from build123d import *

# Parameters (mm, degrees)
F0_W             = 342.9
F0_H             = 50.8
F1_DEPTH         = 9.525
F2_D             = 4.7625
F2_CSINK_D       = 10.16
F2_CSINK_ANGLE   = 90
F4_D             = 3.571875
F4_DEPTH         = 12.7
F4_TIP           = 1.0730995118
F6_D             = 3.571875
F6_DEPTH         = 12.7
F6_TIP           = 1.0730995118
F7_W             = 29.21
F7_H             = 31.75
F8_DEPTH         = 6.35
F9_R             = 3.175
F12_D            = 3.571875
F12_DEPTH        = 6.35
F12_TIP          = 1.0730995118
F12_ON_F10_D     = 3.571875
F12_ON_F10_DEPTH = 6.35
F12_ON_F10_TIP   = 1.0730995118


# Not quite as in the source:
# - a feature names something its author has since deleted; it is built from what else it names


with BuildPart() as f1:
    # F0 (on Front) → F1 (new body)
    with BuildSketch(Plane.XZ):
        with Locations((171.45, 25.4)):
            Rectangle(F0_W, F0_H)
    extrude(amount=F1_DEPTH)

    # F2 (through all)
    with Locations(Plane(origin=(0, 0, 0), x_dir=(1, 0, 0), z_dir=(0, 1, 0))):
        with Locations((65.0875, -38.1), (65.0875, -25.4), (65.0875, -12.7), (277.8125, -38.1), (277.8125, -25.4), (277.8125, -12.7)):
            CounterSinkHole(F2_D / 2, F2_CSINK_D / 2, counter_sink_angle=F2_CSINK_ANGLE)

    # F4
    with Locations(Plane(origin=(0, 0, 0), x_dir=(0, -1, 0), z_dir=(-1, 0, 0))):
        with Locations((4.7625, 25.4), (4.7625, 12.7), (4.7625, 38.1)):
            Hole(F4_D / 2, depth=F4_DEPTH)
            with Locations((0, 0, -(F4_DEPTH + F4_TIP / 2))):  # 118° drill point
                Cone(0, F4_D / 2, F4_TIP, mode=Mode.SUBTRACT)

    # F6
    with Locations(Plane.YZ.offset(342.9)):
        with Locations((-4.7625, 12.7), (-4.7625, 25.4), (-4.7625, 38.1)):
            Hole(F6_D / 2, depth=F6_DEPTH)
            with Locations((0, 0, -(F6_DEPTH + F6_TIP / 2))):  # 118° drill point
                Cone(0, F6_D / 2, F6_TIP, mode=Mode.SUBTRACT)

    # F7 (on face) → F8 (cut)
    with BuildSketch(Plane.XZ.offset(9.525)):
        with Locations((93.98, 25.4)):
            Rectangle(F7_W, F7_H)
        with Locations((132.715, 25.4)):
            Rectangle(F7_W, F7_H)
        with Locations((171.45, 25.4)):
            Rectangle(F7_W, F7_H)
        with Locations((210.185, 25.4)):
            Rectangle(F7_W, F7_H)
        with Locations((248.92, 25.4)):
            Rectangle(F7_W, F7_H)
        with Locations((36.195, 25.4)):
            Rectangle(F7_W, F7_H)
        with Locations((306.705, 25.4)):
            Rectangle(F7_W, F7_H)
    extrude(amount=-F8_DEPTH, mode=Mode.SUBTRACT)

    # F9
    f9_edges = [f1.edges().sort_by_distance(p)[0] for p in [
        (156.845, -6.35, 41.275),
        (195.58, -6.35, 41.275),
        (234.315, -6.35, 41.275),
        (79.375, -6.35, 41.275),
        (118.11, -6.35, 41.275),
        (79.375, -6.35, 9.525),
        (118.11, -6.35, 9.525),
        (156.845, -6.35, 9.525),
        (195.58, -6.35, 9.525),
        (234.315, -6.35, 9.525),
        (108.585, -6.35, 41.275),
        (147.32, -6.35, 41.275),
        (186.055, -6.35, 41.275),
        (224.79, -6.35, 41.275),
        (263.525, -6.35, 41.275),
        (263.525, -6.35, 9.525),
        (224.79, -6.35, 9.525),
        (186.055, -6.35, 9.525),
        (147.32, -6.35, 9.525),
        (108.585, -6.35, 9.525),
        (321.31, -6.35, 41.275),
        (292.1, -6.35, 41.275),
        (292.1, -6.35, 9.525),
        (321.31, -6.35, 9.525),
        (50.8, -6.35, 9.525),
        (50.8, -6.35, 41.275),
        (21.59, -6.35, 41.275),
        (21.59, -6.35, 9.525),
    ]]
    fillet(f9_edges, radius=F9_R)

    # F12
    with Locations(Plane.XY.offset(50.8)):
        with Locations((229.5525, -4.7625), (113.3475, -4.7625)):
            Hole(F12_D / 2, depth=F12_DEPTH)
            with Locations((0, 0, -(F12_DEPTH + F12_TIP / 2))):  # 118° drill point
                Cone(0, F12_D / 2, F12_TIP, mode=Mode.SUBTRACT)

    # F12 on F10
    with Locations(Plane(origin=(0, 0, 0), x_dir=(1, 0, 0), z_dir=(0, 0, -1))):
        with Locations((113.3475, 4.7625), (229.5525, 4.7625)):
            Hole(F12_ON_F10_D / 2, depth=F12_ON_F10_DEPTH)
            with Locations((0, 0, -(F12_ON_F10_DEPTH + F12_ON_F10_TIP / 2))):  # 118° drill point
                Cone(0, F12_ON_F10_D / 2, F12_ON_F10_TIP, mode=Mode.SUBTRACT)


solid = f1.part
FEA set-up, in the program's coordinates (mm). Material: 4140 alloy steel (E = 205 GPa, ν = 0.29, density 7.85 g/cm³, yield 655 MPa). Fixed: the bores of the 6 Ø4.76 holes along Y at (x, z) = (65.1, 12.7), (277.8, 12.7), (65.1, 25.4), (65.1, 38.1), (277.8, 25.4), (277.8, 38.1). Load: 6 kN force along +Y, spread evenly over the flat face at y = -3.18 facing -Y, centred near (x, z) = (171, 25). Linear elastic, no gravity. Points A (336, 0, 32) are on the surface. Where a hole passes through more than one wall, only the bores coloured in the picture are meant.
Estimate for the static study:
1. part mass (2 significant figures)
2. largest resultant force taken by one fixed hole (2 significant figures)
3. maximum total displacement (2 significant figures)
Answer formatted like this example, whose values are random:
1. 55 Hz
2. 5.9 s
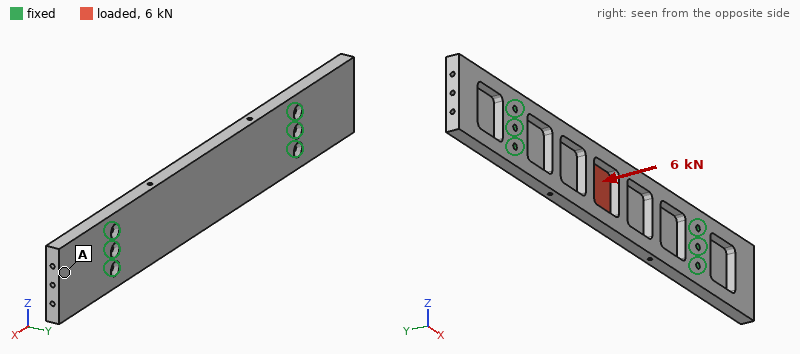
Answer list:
1. 960 g
2. 2.6 kN
3. 0.70 mm
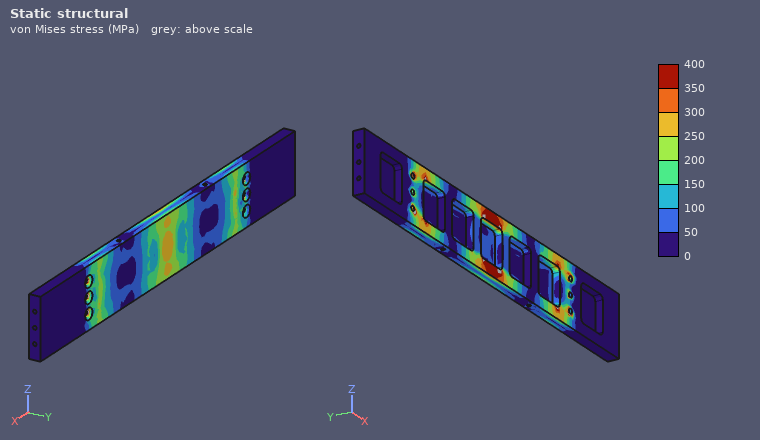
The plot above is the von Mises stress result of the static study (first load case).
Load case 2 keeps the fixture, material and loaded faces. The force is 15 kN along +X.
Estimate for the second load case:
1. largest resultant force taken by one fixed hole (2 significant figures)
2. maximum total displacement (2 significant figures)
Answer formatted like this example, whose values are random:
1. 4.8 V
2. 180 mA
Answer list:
1. 3.1 kN
2. 18 µm
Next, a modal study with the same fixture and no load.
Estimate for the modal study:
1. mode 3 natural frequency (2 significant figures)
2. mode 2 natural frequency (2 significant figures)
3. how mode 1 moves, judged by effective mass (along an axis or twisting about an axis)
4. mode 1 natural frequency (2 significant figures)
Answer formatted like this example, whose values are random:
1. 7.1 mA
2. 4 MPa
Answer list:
1. 1500 Hz
2. 1500 Hz
3. along Y
4. 1000 Hz
